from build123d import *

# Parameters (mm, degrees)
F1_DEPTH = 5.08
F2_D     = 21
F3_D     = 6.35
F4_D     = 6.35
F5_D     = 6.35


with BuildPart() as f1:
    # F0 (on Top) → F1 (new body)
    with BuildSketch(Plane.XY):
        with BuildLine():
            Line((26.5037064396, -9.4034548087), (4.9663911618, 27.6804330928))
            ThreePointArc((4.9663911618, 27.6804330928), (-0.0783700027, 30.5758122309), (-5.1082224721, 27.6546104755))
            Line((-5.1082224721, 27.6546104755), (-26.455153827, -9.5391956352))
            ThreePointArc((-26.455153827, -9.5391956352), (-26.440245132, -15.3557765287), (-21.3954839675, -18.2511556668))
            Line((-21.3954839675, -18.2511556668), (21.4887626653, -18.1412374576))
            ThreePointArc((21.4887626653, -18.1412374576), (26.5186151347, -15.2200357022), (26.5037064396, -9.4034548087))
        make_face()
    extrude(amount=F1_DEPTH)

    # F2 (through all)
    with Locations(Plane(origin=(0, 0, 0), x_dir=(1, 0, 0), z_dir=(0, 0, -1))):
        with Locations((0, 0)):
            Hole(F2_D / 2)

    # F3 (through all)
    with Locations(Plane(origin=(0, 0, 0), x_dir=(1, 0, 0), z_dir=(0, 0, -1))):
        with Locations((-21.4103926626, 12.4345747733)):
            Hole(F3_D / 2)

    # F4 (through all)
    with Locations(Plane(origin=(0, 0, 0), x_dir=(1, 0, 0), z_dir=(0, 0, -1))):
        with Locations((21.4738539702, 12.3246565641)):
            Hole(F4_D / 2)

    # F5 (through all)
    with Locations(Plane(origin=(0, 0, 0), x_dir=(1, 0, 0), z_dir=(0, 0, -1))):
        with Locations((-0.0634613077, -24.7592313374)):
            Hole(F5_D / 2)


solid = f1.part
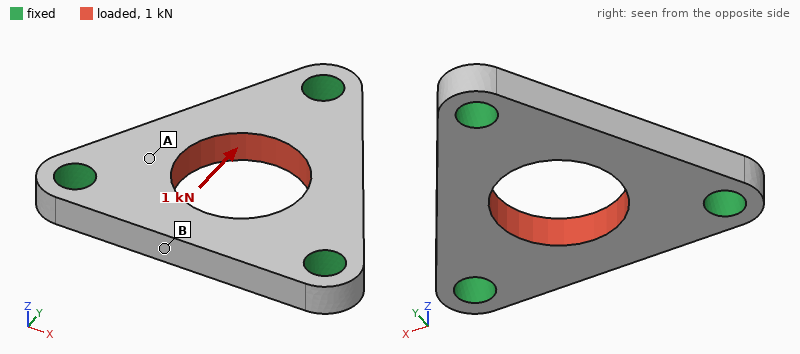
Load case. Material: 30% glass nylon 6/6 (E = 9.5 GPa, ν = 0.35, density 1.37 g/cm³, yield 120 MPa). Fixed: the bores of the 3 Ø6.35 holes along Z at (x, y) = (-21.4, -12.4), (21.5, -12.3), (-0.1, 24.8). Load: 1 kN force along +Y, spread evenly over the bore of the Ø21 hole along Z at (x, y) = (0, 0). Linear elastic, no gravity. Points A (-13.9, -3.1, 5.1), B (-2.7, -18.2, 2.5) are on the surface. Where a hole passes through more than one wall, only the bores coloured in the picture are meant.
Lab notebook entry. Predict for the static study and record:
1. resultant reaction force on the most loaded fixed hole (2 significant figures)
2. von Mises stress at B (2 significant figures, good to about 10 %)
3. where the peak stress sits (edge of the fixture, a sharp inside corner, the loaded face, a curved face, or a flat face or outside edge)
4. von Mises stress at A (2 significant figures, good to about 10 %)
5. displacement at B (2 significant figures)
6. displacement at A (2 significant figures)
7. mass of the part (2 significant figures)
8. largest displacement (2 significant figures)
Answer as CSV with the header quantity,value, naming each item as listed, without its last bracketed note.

quantity,value
resultant reaction force on the most loaded fixed hole,350 N
von Mises stress at B,10 MPa
where the peak stress sits,edge of the fixture
von Mises stress at A,3.5 MPa
displacement at B,29 µm
displacement at A,16 µm
mass of the part,8.4 g
largest displacement,33 µm
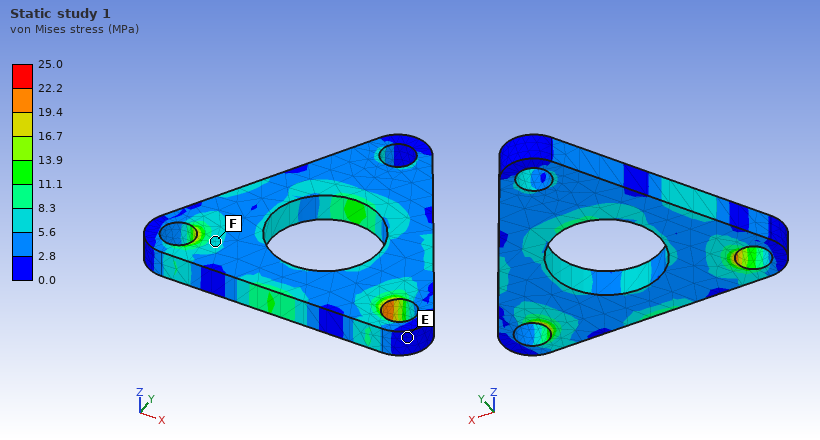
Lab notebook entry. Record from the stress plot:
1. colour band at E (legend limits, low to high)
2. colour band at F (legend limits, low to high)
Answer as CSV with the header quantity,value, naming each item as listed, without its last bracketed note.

quantity,value
colour band at E,0.0 to 2.8 MPa
colour band at F,5.6 to 8.3 MPa
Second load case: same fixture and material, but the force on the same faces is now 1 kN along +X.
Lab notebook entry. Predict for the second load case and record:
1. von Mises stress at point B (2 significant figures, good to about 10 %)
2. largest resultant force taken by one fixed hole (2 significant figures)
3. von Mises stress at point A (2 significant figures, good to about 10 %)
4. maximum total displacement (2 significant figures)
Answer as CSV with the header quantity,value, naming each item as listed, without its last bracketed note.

quantity,value
von Mises stress at point B,3.1 MPa
largest resultant force taken by one fixed hole,340 N
von Mises stress at point A,5.6 MPa
maximum total displacement,29 µm
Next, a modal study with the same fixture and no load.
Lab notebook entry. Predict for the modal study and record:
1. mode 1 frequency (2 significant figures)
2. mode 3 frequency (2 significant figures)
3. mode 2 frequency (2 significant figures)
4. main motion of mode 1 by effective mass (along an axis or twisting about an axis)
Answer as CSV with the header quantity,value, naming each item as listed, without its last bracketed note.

quantity,value
mode 1 frequency,8800 Hz
mode 3 frequency,9400 Hz
mode 2 frequency,9400 Hz
main motion of mode 1 by effective mass,along Z
